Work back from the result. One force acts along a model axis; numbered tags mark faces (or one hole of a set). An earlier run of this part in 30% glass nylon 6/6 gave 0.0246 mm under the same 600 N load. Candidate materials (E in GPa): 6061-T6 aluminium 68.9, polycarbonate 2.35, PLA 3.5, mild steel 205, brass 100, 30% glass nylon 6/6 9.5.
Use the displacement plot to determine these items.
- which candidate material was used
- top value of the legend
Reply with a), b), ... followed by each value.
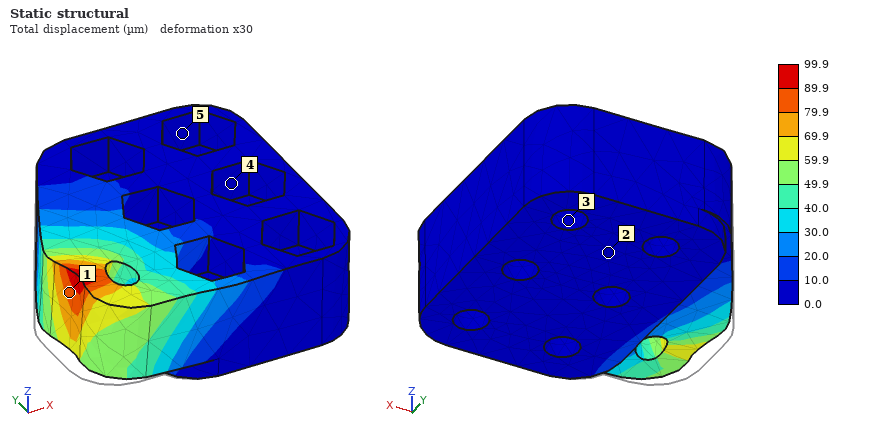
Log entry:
a) polycarbonate
b) 99.9 µm
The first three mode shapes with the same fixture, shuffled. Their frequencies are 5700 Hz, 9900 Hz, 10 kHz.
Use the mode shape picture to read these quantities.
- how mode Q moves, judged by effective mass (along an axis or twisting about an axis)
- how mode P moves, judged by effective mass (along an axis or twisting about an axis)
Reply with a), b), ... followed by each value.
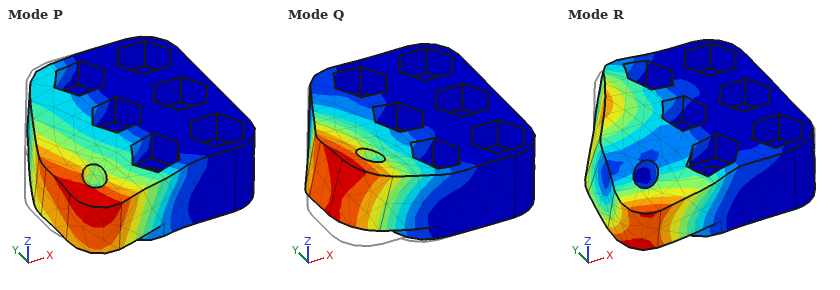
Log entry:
a) along Z
b) along Y
